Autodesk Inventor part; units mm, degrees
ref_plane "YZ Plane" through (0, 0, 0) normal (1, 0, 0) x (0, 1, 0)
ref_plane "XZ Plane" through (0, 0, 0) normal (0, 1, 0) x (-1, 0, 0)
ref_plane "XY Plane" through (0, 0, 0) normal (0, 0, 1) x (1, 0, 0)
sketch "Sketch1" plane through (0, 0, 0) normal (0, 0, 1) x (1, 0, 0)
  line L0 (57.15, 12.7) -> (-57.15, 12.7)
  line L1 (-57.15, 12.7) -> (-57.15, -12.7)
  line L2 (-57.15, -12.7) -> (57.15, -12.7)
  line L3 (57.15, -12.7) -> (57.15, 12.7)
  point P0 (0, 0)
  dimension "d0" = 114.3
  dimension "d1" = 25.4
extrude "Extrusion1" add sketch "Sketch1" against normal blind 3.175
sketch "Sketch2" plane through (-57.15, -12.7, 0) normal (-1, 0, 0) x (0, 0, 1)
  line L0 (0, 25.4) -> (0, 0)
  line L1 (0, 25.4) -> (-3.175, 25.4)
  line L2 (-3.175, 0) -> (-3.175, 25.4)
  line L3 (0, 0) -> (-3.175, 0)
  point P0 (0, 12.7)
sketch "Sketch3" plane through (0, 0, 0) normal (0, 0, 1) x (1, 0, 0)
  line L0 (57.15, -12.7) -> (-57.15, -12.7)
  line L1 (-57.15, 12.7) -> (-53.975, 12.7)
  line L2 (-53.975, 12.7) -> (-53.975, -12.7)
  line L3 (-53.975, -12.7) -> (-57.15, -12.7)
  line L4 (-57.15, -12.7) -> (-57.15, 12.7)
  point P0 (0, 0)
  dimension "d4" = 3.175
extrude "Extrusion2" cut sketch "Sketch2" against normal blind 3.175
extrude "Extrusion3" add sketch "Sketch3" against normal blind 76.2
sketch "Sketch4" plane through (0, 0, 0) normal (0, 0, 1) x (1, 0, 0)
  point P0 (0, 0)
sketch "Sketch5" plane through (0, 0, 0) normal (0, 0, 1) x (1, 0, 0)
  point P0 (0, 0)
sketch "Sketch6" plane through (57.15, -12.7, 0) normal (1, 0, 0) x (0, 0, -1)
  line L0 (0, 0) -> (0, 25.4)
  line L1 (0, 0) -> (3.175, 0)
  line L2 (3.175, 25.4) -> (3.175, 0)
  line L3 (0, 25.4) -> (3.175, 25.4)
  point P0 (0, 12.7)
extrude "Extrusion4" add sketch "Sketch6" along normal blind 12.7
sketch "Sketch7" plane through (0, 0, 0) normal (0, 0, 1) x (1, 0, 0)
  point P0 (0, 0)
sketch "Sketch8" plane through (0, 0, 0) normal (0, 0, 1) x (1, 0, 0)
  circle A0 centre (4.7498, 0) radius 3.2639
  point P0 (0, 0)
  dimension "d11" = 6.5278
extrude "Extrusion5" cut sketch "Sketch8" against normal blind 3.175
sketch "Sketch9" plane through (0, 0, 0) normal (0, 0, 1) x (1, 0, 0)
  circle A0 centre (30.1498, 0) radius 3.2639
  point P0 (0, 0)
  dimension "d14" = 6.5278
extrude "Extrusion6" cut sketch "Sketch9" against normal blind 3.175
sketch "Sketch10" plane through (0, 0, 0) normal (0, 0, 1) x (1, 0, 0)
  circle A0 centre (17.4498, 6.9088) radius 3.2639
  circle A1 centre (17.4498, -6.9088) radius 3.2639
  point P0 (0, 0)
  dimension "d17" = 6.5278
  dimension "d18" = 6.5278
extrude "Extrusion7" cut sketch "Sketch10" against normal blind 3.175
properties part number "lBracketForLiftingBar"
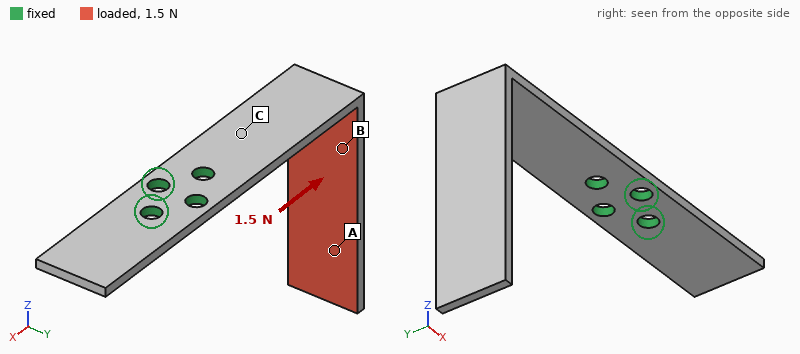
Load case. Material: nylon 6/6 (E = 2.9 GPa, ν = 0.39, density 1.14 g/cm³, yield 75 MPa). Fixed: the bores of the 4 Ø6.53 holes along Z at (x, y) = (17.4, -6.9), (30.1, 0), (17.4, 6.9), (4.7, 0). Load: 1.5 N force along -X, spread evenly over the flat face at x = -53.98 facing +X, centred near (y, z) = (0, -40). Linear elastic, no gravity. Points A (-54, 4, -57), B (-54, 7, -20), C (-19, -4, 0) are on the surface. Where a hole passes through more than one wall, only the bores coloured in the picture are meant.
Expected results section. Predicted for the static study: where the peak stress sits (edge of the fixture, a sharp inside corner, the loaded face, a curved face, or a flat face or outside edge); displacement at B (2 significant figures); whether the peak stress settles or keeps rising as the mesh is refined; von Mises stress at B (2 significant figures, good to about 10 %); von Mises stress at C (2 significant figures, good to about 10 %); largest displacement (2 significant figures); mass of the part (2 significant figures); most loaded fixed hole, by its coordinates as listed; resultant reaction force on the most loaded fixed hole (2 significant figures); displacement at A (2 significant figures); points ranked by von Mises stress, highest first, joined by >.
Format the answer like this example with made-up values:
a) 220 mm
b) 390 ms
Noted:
a) edge of the fixture
b) 0.56 mm
c) keeps rising
d) 0.74 MPa
e) 1.3 MPa
f) 1.7 mm
g) 18 g
h) (4.7, 0)
i) 2.0 N
j) 1.2 mm
k) C > B > A
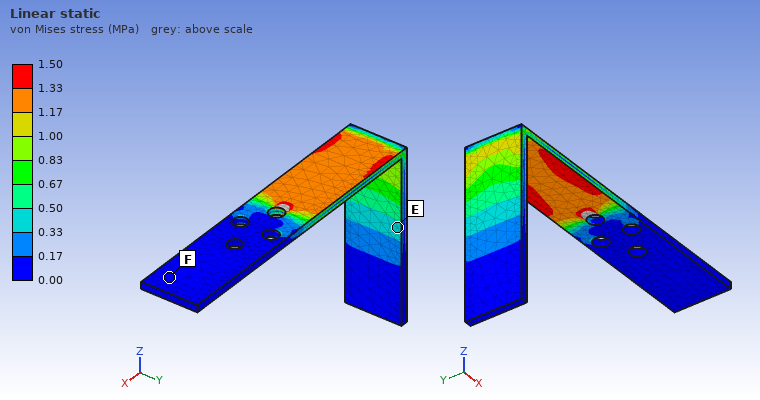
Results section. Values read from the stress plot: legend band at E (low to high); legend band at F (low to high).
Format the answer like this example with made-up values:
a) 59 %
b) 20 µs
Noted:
a) 0.33 to 0.50 MPa
b) 0.00 to 0.17 MPa
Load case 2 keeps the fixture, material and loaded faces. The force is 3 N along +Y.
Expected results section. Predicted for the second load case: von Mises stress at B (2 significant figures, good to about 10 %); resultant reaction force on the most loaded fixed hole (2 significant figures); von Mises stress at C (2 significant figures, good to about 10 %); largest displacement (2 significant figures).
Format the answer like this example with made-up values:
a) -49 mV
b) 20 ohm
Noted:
a) 0.28 MPa
b) 6.2 N
c) 2.4 MPa
d) 1.8 mm
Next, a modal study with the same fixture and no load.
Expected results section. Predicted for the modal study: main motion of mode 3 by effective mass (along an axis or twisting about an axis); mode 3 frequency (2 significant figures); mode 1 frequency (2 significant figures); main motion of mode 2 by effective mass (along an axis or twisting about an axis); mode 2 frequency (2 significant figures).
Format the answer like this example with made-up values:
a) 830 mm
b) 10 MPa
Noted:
a) along Z
b) 180 Hz
c) 62 Hz
d) along Y
e) 96 Hz
